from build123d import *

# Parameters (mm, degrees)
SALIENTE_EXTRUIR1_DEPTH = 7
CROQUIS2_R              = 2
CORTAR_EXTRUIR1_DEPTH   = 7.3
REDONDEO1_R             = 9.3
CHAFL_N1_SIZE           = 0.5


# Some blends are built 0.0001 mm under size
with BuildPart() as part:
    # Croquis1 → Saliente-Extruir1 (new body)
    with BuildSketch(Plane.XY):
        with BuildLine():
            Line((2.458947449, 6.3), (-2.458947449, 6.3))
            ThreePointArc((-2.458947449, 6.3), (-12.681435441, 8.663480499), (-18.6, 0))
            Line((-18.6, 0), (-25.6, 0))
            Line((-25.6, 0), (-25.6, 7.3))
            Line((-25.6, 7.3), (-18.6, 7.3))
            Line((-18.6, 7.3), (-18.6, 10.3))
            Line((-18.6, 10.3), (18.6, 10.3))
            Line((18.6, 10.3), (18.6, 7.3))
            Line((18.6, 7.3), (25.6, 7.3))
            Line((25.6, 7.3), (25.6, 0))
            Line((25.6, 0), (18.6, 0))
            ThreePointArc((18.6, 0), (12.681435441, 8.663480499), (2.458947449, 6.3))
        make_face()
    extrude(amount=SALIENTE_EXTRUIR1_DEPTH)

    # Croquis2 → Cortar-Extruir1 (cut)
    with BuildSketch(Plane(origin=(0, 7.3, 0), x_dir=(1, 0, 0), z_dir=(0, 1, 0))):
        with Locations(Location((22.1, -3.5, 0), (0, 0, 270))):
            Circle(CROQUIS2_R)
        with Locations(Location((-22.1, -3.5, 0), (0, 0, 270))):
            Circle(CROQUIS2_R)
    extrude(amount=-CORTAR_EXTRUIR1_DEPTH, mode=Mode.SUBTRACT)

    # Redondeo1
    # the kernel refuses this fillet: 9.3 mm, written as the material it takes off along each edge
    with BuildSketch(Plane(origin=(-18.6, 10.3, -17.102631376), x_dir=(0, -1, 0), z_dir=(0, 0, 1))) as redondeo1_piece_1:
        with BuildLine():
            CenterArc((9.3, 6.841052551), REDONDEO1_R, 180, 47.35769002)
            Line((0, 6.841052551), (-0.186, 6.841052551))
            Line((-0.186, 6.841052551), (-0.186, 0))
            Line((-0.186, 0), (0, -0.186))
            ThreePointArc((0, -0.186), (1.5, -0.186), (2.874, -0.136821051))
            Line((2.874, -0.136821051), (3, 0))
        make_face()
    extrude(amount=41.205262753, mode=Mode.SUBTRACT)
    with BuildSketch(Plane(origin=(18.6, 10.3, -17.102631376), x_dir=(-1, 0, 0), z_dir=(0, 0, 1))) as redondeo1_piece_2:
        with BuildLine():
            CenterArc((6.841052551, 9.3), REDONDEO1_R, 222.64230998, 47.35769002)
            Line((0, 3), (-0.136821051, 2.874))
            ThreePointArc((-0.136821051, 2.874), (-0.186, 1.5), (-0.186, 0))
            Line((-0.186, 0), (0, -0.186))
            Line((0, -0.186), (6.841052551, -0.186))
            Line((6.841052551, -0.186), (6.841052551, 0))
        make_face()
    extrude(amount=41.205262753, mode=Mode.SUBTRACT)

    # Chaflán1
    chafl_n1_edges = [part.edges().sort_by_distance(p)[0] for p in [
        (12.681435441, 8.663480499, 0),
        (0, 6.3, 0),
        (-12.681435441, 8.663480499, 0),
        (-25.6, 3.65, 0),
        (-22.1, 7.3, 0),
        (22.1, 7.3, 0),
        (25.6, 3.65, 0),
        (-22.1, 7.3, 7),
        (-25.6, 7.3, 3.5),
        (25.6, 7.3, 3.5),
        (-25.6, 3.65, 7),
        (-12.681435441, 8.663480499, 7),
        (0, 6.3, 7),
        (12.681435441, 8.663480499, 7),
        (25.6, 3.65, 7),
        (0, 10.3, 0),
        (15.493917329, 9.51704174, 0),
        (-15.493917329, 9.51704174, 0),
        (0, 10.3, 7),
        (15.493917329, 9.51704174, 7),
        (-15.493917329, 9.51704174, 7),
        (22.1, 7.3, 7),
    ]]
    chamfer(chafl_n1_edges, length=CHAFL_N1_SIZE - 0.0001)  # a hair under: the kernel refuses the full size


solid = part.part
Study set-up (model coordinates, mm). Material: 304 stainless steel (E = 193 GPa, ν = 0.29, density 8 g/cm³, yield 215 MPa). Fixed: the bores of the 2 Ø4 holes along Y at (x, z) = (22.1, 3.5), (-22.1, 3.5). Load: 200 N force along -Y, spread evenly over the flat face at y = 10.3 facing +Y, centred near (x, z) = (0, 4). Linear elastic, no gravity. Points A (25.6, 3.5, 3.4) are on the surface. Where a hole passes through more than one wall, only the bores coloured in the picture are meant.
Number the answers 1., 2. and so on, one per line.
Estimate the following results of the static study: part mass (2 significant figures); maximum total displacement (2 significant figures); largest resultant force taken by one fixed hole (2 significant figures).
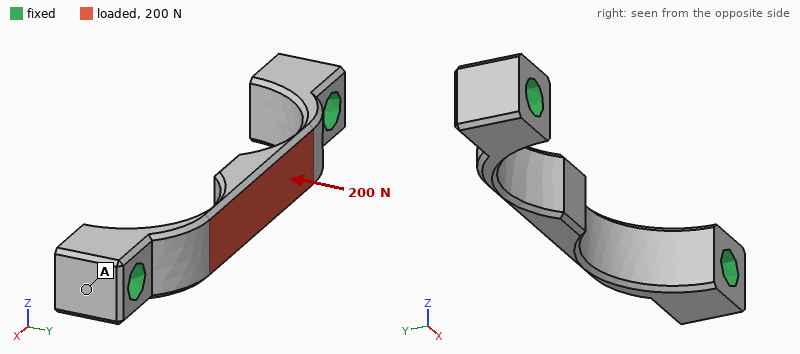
1. 9.0 g
2. 28 µm
3. 210 N
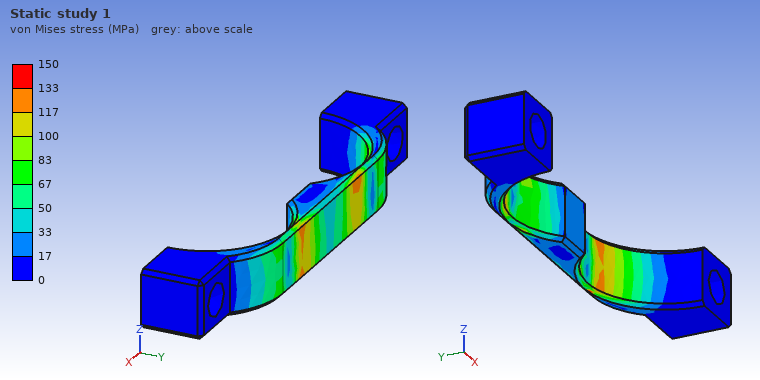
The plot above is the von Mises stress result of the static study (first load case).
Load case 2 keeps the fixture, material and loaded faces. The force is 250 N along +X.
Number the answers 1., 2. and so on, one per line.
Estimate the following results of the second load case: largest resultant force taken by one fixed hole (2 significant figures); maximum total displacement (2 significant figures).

1. 130 N
2. 5.9 µm
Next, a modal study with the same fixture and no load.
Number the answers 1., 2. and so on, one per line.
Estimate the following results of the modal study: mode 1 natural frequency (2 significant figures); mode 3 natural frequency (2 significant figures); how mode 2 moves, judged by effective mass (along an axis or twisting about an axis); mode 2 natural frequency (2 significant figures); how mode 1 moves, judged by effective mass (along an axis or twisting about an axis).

1. 7800 Hz
2. 14 kHz
3. along Z
4. 10 kHz
5. along Y
